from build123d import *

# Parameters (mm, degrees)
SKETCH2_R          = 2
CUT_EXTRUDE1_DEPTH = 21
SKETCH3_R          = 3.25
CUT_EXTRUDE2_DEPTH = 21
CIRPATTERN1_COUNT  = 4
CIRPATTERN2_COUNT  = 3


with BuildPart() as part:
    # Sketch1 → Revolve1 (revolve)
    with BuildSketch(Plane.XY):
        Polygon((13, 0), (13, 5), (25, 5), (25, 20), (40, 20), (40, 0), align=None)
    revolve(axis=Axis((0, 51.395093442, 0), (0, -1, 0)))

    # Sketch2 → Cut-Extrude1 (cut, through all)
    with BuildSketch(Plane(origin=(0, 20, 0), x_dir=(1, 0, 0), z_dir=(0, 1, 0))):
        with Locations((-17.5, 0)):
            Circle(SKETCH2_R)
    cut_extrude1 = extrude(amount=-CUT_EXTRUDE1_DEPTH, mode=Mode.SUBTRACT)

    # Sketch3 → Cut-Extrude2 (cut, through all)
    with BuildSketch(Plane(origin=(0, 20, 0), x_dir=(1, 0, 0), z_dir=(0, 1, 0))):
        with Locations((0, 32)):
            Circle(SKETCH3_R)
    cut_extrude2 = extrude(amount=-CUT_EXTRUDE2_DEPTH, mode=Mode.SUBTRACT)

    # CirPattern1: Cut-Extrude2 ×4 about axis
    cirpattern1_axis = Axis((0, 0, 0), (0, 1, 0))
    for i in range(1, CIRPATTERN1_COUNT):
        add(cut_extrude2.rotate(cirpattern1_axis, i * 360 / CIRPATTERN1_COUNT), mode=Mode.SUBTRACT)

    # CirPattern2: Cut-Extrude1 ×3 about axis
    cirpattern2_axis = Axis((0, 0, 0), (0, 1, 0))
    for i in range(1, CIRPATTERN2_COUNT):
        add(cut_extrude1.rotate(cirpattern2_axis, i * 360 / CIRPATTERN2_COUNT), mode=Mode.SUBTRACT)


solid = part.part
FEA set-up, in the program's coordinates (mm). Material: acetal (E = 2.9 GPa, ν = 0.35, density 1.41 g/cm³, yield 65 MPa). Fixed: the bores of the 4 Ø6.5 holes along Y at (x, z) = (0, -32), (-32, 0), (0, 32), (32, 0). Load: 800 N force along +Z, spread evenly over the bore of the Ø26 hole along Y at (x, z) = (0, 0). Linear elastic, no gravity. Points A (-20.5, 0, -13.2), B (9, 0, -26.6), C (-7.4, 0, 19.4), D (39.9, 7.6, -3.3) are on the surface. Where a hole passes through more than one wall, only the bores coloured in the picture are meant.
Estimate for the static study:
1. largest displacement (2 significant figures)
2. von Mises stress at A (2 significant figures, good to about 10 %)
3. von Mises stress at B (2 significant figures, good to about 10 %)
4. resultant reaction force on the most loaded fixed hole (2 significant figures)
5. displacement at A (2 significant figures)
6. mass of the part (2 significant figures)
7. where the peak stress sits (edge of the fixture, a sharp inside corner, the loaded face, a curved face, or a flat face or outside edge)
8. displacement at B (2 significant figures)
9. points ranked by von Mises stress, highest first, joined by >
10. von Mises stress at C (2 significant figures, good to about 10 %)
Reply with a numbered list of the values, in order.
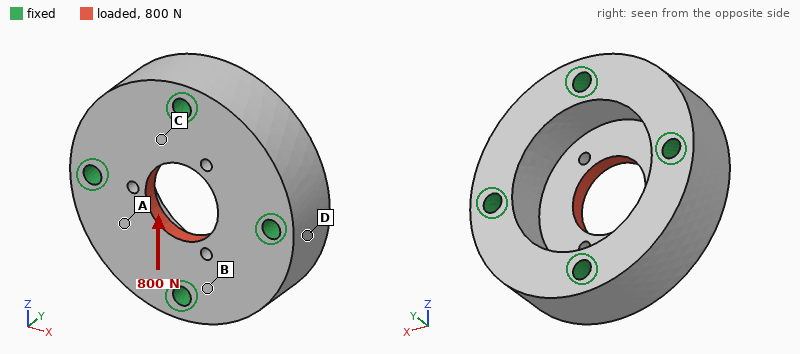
1. 21 µm
2. 0.72 MPa
3. 1.2 MPa
4. 220 N
5. 8.7 µm
6. 92 g
7. a curved face
8. 7.0 µm
9. C > B > A > D
10. 1.9 MPa
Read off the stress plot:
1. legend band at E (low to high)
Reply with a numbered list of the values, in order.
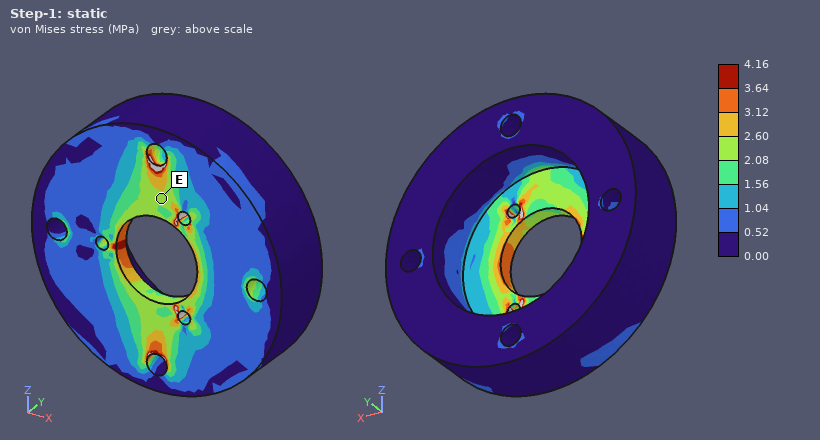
1. 2.08 to 2.60 MPa
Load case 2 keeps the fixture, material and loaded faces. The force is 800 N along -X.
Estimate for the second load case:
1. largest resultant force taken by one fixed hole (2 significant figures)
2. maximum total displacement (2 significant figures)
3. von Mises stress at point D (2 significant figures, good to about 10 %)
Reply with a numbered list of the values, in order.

1. 220 N
2. 21 µm
3. 0.46 MPa
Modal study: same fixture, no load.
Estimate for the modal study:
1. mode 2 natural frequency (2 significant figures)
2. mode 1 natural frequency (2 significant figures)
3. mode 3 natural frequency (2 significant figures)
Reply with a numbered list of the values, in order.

1. 6300 Hz
2. 6200 Hz
3. 6500 Hz
